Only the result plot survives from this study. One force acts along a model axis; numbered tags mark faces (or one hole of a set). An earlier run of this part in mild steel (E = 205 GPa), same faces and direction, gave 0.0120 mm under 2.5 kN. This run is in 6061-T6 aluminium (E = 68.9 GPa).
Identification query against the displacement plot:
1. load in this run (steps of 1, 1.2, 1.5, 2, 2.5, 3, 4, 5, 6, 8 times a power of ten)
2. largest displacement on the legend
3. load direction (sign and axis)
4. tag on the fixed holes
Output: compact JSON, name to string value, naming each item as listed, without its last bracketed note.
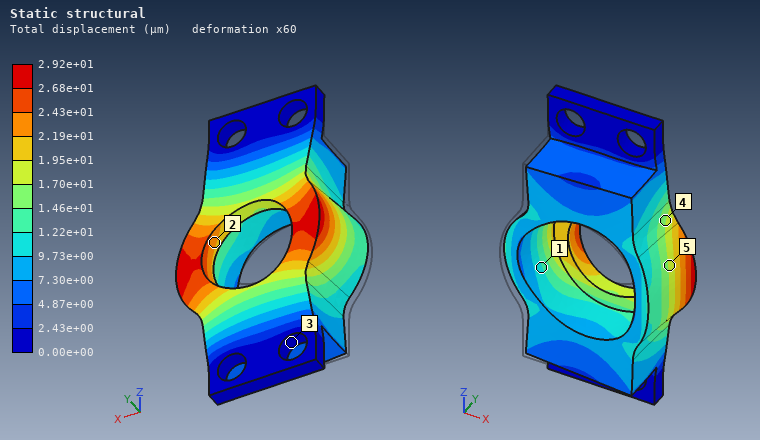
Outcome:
{"load in this run": "2 kN", "largest displacement on the legend": "2.92e+01 µm", "load direction": "+X", "tag on the fixed holes": "3"}
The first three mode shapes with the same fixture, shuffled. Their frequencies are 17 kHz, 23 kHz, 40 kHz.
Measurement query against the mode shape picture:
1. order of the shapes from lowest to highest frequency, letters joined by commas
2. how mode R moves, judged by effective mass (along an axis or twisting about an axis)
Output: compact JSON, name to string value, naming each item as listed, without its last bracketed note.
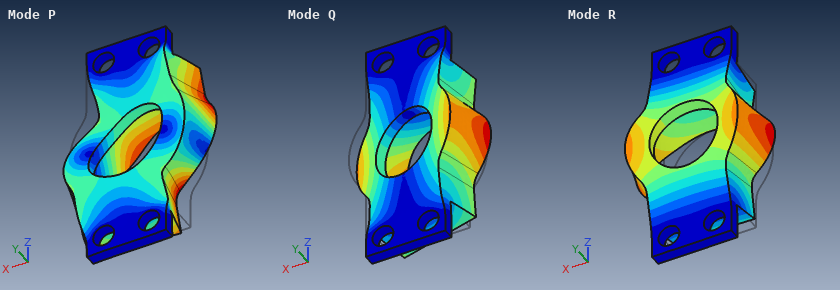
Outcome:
{"order of the shapes from lowest to highest frequency, letters joined by commas": "R, Q, P", "how mode R moves, judged by effective mass": "along Y"}
